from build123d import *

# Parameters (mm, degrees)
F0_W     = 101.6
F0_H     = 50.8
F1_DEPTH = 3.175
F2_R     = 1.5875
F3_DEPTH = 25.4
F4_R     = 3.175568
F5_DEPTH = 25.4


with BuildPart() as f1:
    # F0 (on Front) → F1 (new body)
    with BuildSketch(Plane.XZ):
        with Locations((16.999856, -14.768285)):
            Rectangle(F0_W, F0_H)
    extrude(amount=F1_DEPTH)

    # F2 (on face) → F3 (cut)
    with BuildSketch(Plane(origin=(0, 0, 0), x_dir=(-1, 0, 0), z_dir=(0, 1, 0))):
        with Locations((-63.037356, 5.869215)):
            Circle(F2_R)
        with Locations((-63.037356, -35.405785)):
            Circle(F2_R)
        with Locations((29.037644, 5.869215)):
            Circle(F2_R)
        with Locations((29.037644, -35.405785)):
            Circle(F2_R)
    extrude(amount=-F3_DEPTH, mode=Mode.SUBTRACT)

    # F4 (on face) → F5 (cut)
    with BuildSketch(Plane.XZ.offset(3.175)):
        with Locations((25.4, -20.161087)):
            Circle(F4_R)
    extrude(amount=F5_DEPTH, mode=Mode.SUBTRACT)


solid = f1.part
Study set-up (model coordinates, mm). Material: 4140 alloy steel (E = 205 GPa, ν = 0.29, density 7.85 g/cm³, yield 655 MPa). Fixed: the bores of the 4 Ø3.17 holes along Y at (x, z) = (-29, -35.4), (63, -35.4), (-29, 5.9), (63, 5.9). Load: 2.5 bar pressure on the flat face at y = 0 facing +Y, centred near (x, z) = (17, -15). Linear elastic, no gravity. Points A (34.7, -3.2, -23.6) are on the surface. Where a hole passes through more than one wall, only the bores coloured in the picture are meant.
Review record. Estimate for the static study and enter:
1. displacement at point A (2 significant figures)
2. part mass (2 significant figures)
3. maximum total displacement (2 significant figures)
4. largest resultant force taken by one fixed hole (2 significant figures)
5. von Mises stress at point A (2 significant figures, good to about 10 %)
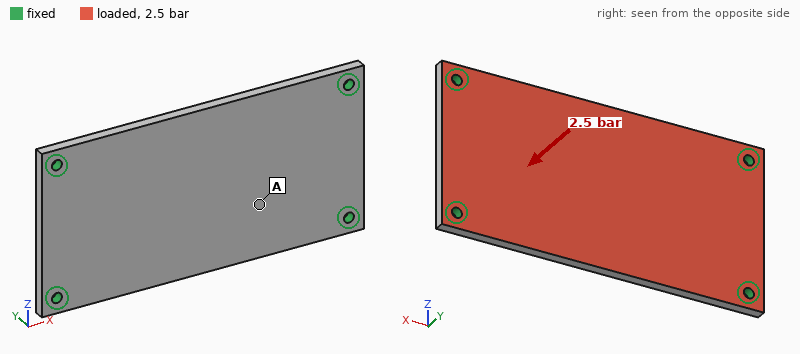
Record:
0.084 mm
130 g
0.11 mm
320 N
34 MPa
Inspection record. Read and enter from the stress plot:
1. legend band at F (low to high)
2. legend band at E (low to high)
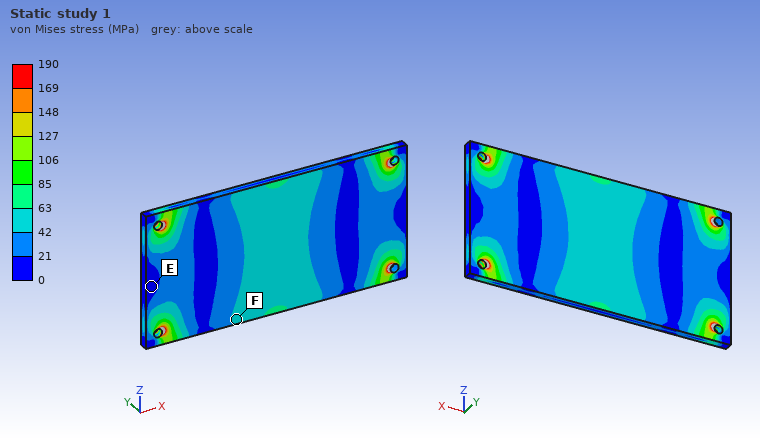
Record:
42 to 63 MPa
0 to 21 MPa
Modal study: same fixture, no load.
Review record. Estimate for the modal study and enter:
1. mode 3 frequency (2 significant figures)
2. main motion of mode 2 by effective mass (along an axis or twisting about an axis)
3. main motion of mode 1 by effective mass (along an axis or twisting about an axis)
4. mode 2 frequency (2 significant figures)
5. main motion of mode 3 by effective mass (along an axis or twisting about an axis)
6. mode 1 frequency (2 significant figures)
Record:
4700 Hz
twisting about X
along Y
3000 Hz
twisting about Z
1700 Hz
